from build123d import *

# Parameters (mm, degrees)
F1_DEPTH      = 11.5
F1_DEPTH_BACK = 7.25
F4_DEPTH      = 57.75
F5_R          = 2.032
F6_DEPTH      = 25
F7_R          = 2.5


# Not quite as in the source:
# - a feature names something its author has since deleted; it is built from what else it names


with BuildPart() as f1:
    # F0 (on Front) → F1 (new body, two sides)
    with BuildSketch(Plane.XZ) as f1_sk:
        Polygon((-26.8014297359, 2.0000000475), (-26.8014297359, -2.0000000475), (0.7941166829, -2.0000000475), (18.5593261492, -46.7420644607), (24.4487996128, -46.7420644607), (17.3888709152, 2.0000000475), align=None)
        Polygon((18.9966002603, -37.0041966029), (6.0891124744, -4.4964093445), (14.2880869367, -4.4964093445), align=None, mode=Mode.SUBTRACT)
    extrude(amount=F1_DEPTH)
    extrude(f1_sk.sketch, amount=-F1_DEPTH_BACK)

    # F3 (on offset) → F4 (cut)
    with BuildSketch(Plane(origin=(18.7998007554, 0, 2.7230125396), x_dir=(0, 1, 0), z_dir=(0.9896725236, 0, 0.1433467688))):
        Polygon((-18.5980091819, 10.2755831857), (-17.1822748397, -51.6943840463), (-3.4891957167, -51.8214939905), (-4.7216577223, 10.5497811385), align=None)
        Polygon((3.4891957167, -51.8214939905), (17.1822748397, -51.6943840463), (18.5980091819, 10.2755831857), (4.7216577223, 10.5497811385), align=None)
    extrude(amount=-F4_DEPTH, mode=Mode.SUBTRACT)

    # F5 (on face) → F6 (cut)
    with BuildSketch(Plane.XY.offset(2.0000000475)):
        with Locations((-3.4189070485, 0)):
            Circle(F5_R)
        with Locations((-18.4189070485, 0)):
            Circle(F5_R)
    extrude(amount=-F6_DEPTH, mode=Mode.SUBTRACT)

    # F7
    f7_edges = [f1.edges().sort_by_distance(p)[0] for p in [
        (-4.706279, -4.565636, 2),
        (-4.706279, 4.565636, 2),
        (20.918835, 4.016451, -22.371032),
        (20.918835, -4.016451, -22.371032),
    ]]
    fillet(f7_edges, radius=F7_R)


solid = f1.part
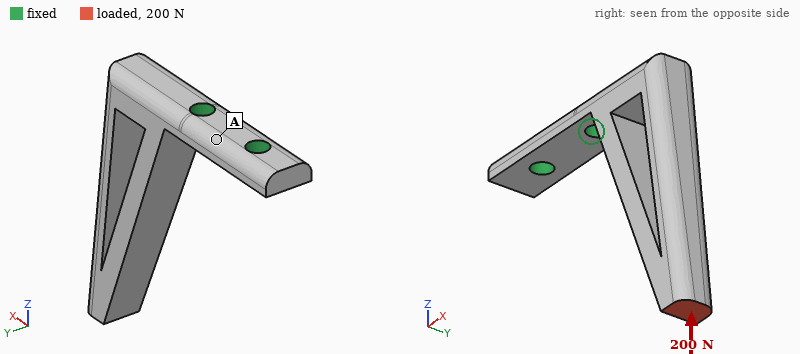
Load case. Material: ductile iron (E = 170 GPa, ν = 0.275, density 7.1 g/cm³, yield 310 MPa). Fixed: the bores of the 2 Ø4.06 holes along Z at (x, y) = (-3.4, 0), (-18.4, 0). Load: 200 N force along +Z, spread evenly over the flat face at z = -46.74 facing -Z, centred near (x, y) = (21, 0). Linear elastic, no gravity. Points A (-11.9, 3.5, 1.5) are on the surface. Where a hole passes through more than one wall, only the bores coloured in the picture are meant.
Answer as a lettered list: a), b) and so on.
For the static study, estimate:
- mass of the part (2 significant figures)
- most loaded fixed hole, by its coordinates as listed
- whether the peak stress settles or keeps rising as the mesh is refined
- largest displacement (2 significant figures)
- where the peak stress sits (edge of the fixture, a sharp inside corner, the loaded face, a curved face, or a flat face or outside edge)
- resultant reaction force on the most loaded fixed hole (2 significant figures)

a) 31 g
b) (-3.4, 0)
c) keeps rising
d) 0.18 mm
e) edge of the fixture
f) 210 N
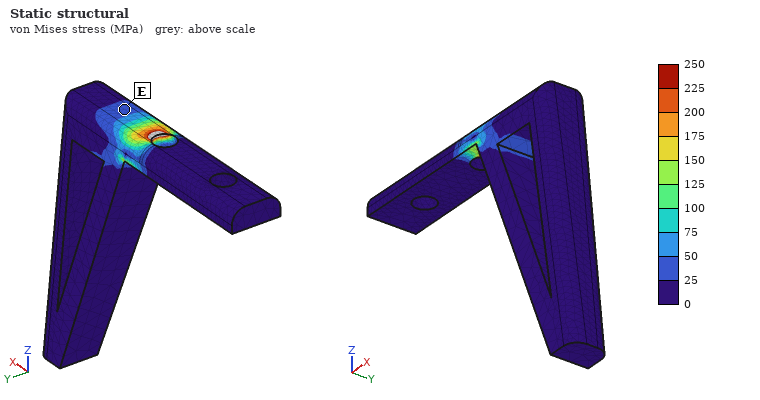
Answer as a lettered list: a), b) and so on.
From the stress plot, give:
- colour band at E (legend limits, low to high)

a) 25 to 50 MPa
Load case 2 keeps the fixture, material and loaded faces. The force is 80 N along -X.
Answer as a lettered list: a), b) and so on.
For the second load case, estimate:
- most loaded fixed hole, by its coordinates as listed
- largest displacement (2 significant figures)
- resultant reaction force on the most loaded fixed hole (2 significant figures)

a) (-3.4, 0)
b) 0.16 mm
c) 61 N
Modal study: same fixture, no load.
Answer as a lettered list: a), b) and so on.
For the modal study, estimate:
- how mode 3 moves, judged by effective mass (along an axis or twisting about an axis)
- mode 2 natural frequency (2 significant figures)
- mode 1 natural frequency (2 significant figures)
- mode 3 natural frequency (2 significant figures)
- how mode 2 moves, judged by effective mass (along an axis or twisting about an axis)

a) along Y
b) 1600 Hz
c) 1300 Hz
d) 7400 Hz
e) along Y
